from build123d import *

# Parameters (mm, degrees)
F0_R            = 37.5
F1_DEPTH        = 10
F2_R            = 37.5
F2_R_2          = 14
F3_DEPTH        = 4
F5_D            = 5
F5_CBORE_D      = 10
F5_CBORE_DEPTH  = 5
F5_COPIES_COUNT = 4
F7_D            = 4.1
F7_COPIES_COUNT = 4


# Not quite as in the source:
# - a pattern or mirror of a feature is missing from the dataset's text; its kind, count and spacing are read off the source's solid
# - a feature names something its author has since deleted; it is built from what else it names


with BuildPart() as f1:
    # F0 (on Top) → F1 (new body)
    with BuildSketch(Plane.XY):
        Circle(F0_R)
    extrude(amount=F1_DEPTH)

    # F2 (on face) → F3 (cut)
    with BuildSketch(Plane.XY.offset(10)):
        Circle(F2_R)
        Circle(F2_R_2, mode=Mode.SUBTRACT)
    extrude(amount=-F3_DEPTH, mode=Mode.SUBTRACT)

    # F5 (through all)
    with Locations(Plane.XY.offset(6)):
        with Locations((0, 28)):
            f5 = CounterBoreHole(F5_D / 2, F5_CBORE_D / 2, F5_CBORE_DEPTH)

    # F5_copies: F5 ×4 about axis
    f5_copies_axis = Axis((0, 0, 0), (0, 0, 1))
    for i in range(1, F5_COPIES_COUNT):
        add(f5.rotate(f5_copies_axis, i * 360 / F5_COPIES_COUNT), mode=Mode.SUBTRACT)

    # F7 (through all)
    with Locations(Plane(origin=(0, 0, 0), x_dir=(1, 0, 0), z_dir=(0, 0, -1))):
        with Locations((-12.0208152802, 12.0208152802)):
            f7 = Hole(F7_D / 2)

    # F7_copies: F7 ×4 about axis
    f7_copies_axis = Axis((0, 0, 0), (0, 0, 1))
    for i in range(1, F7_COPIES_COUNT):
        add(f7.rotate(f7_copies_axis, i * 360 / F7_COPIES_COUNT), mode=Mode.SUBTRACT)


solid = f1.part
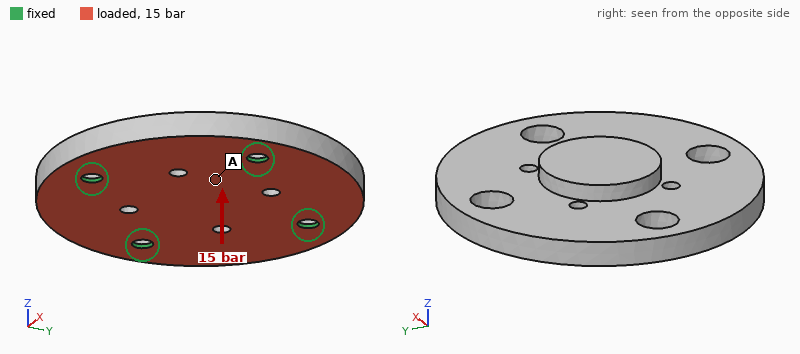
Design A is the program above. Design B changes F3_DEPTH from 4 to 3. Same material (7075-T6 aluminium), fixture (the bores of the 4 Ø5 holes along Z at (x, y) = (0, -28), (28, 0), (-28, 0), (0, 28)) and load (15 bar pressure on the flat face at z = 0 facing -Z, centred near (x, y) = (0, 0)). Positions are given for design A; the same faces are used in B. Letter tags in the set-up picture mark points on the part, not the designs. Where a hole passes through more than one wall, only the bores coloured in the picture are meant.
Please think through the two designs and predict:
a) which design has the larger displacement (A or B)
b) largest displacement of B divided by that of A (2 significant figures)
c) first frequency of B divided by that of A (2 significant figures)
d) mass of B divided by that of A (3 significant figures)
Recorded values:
A
0.83
1.0
1.13
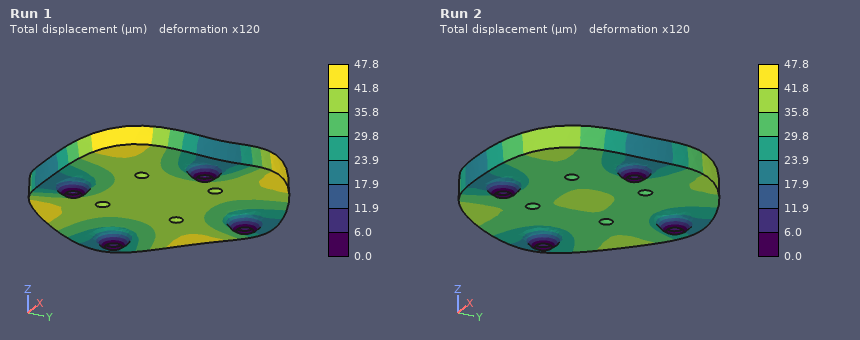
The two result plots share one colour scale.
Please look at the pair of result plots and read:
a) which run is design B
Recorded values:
Run 2
